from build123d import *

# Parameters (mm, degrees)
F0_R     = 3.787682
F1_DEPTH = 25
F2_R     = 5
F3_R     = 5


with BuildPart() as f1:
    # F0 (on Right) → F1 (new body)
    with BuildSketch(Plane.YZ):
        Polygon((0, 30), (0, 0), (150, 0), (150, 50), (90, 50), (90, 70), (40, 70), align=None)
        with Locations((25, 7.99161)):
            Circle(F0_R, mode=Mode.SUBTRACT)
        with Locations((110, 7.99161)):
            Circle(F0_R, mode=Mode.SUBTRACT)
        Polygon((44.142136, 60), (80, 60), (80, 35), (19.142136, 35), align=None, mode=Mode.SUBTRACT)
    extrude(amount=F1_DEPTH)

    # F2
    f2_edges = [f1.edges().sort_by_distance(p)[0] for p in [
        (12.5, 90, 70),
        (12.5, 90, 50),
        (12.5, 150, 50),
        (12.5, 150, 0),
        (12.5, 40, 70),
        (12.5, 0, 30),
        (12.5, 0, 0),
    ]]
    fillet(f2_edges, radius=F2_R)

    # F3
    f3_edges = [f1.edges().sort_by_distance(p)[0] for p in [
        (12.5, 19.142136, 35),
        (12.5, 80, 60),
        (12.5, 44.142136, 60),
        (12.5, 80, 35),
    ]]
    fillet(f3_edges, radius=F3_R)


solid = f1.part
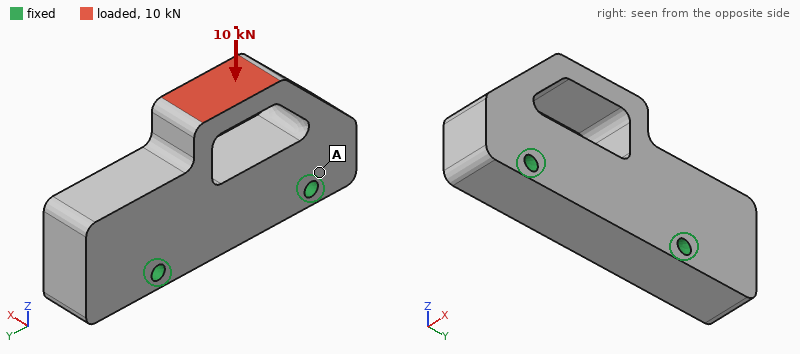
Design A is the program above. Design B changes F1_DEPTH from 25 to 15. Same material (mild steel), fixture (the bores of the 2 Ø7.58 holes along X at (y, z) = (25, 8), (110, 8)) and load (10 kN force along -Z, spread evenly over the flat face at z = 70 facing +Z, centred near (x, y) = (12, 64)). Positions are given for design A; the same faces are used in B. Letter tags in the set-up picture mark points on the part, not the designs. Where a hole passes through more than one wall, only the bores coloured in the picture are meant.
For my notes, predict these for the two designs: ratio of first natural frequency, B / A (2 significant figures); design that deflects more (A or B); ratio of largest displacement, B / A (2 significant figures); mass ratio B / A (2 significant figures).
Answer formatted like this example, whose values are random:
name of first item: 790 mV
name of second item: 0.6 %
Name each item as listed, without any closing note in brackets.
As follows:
ratio of first natural frequency, B / A: 0.70
design that deflects more: B
ratio of largest displacement, B / A: 1.6
mass ratio B / A: 0.60
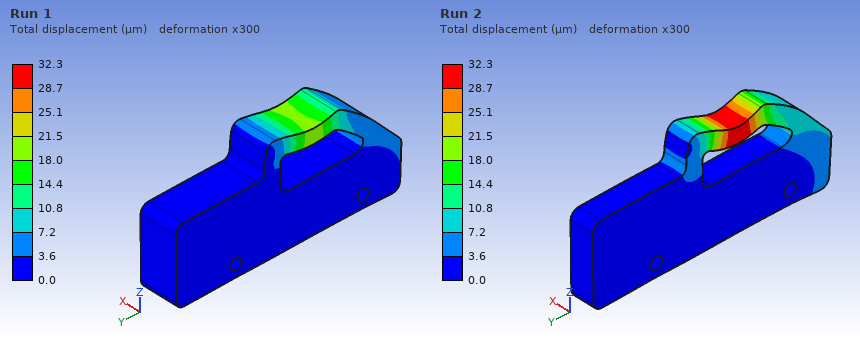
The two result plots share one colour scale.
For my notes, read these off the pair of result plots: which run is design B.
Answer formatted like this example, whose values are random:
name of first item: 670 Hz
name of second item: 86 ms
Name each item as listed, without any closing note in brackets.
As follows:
which run is design B: Run 2
